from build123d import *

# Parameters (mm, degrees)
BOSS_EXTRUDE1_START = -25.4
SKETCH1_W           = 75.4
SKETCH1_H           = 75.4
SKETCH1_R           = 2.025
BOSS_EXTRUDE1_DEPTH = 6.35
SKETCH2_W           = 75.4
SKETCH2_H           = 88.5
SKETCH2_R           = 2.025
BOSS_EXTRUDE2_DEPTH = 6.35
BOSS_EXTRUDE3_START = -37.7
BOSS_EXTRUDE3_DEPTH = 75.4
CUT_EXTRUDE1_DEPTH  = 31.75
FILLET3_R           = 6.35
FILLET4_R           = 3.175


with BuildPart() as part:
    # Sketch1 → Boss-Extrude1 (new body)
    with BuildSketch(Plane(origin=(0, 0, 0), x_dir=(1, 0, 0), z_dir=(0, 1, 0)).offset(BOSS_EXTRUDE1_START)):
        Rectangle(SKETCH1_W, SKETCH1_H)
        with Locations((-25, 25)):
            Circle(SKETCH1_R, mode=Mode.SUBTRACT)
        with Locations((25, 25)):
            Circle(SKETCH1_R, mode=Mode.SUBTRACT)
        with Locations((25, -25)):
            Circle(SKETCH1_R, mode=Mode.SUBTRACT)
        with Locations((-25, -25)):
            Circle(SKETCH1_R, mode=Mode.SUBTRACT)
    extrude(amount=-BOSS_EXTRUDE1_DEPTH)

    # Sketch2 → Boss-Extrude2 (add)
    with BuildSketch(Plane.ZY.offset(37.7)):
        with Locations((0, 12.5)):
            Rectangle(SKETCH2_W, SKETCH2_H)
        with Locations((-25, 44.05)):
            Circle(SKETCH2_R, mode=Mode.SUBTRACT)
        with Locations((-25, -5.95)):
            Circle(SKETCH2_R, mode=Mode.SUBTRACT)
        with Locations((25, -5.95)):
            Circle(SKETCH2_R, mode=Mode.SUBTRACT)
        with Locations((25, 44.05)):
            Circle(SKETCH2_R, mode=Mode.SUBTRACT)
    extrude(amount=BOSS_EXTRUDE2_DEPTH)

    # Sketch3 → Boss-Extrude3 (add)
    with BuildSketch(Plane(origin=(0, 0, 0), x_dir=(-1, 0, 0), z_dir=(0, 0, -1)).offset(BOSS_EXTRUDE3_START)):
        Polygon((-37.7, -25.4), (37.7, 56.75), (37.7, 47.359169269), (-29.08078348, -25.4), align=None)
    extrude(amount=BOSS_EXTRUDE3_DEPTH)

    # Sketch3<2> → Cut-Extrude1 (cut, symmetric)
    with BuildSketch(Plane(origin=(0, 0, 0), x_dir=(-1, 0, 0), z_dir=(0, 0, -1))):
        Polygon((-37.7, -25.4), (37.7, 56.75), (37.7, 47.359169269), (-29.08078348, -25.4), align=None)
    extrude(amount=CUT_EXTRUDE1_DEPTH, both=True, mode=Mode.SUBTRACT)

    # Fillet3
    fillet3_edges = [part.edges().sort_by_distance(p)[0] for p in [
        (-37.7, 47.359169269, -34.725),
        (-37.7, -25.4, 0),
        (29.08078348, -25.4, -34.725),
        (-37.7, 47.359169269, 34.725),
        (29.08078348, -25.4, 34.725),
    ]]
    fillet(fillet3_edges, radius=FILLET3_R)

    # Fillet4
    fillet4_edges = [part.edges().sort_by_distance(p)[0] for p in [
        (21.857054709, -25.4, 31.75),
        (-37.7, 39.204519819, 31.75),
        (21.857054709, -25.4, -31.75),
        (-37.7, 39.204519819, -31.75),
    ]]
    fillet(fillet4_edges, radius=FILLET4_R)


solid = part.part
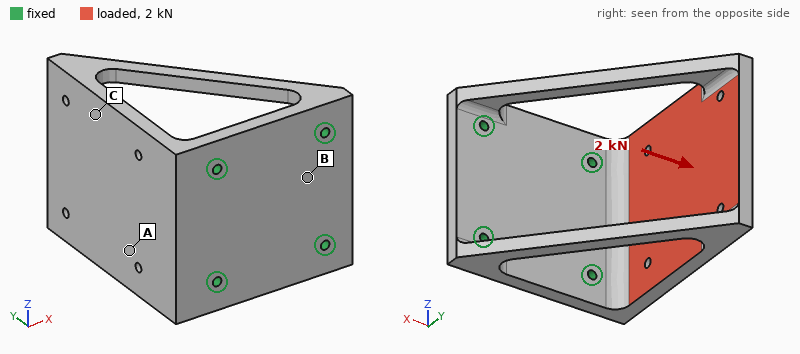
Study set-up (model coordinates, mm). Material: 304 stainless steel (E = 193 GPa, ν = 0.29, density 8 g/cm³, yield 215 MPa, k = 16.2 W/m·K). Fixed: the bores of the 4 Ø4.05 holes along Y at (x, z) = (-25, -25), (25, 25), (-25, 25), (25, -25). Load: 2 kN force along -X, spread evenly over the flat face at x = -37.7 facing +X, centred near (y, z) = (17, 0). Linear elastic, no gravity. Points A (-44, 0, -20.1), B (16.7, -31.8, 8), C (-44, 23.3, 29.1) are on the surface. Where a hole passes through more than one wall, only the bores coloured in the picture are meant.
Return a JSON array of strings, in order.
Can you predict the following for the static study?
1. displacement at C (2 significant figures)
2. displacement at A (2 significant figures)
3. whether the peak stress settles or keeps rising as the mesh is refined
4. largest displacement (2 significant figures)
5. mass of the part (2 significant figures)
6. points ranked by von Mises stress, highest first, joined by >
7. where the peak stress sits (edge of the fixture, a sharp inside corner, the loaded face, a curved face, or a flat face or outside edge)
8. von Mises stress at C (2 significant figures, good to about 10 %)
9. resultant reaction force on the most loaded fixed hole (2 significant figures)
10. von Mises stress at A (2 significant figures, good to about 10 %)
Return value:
["54 µm", "41 µm", "keeps rising", "63 µm", "700 g", "C > A > B", "edge of the fixture", "27 MPa", "800 N", "16 MPa"]
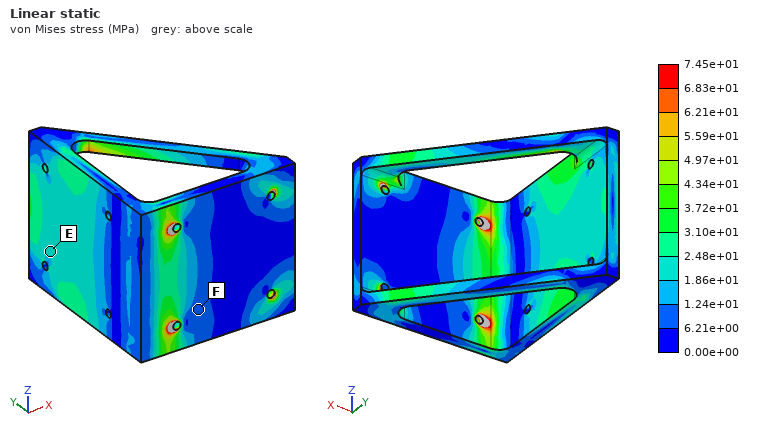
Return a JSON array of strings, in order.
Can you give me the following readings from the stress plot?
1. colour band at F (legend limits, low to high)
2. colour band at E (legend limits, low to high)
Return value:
["6.21e+00 to 1.24e+01 MPa", "1.86e+01 to 2.48e+01 MPa"]
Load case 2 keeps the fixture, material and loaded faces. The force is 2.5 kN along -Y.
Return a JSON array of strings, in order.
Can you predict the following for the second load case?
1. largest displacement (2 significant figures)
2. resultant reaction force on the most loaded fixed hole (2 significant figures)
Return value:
["24 µm", "1.4 kN"]
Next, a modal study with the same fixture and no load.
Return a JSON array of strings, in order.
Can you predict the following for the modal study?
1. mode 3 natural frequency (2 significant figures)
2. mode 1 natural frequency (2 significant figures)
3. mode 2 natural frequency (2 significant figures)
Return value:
["3000 Hz", "1700 Hz", "1700 Hz"]
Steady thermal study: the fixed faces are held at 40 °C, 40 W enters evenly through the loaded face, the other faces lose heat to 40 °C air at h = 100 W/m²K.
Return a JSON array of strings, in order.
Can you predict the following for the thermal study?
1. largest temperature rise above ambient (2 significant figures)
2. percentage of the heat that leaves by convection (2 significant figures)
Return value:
["47 K", "90 %"]
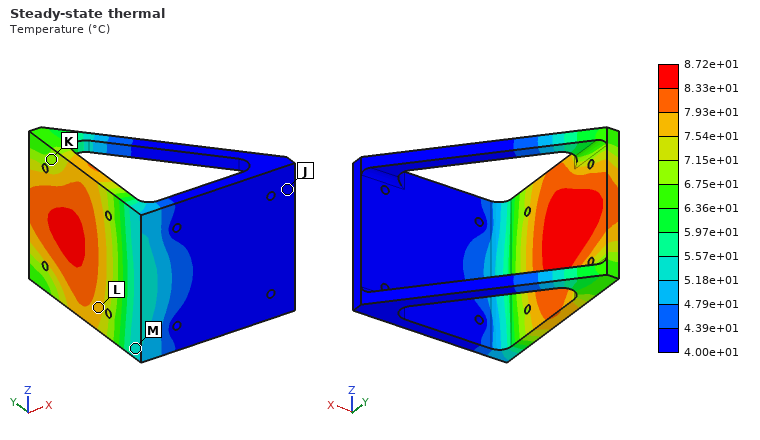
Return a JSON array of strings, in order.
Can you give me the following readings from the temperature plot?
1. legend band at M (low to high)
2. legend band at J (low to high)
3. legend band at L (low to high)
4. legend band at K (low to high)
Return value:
["5.18e+01 to 5.57e+01 °C", "4.00e+01 to 4.39e+01 °C", "7.54e+01 to 7.93e+01 °C", "6.75e+01 to 7.15e+01 °C"]
